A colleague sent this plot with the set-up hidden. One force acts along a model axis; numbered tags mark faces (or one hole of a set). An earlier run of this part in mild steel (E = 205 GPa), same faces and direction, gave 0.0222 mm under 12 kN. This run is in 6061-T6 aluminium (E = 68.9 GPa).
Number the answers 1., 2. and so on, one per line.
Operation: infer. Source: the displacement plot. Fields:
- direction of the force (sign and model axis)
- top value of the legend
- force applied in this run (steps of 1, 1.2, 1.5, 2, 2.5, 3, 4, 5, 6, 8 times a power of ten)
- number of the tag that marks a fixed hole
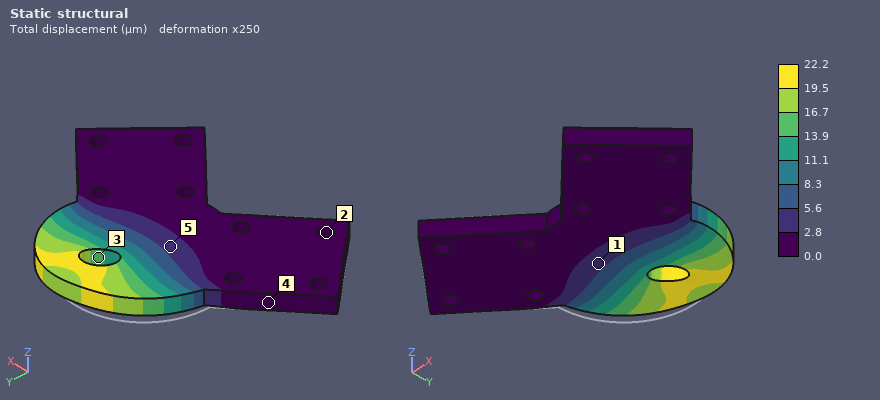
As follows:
1. +X
2. 22.2 µm
3. 4 kN
4. 2
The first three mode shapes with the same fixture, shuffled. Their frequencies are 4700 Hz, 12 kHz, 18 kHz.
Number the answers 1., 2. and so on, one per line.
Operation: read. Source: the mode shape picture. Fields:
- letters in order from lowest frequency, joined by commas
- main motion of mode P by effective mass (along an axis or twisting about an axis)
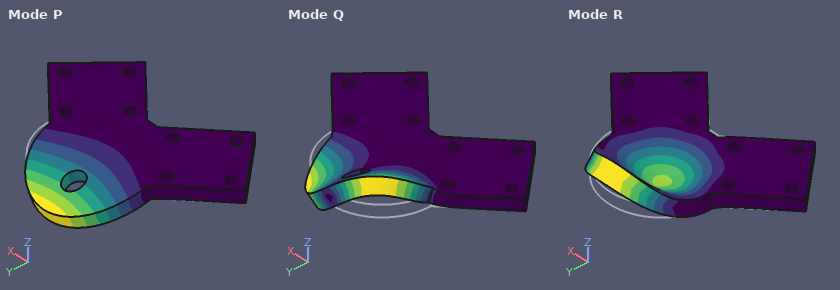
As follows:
1. P, Q, R
2. along Z
